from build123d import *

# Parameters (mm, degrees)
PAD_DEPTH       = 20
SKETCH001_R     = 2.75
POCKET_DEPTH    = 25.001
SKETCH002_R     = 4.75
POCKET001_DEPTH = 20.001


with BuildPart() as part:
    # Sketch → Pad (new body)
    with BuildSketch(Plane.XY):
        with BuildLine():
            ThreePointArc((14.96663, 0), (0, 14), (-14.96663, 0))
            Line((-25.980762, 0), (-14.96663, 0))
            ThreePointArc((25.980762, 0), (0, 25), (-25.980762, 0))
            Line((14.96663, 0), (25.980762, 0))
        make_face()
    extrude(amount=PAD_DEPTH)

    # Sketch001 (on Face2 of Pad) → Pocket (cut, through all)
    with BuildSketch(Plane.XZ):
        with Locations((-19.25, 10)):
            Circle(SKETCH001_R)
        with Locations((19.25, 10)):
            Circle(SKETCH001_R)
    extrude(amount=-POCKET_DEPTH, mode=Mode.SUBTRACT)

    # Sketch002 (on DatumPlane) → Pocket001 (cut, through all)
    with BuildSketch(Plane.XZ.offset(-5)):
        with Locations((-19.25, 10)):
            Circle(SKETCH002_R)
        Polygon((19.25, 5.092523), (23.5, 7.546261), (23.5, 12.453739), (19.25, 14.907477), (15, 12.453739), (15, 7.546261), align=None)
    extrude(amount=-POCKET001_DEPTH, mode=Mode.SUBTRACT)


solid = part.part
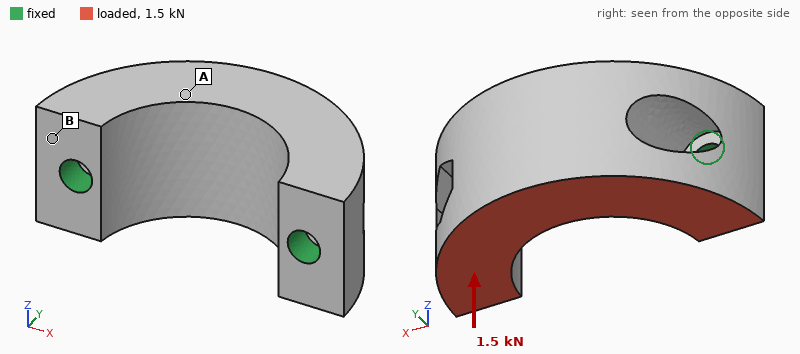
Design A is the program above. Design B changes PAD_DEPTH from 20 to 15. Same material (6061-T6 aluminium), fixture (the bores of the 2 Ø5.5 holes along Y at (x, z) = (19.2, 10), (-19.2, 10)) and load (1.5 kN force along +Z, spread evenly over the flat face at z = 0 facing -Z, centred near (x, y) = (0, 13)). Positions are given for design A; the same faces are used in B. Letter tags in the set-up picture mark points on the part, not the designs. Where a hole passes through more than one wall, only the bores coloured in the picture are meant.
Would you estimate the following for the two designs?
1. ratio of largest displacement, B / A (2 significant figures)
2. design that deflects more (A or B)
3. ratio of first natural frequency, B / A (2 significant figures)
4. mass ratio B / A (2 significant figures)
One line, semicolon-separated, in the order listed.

1.4; B; 1.0; 0.71
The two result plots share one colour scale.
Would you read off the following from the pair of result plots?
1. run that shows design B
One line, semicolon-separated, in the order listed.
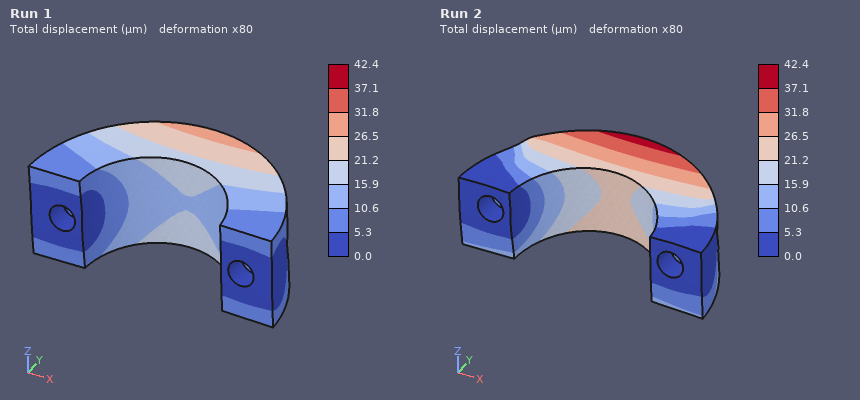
Run 2
